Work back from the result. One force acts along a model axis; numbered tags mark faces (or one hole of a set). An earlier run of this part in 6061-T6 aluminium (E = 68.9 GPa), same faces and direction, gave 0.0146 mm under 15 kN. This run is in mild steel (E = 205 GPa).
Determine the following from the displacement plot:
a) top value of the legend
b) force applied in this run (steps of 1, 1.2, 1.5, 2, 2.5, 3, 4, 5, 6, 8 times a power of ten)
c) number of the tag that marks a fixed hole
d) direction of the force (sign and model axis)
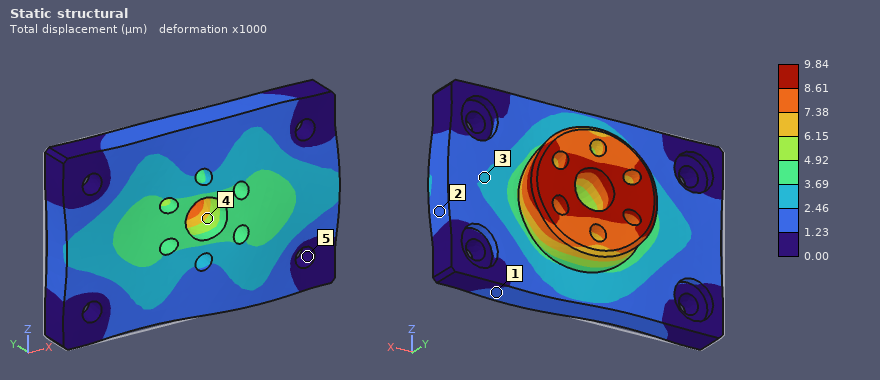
9.84 µm
30 kN
5
+X
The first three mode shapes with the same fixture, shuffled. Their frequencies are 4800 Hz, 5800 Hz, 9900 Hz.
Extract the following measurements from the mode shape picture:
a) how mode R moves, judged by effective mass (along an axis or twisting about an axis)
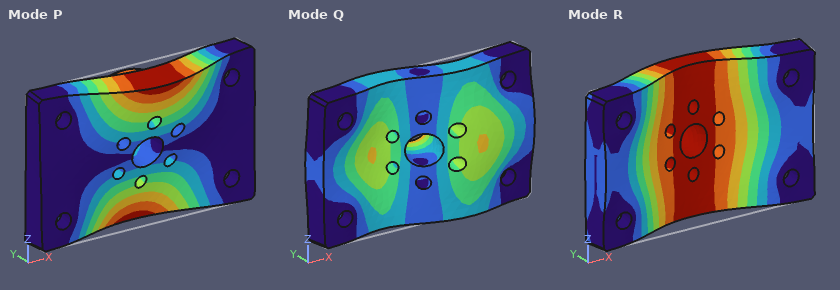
along Y
